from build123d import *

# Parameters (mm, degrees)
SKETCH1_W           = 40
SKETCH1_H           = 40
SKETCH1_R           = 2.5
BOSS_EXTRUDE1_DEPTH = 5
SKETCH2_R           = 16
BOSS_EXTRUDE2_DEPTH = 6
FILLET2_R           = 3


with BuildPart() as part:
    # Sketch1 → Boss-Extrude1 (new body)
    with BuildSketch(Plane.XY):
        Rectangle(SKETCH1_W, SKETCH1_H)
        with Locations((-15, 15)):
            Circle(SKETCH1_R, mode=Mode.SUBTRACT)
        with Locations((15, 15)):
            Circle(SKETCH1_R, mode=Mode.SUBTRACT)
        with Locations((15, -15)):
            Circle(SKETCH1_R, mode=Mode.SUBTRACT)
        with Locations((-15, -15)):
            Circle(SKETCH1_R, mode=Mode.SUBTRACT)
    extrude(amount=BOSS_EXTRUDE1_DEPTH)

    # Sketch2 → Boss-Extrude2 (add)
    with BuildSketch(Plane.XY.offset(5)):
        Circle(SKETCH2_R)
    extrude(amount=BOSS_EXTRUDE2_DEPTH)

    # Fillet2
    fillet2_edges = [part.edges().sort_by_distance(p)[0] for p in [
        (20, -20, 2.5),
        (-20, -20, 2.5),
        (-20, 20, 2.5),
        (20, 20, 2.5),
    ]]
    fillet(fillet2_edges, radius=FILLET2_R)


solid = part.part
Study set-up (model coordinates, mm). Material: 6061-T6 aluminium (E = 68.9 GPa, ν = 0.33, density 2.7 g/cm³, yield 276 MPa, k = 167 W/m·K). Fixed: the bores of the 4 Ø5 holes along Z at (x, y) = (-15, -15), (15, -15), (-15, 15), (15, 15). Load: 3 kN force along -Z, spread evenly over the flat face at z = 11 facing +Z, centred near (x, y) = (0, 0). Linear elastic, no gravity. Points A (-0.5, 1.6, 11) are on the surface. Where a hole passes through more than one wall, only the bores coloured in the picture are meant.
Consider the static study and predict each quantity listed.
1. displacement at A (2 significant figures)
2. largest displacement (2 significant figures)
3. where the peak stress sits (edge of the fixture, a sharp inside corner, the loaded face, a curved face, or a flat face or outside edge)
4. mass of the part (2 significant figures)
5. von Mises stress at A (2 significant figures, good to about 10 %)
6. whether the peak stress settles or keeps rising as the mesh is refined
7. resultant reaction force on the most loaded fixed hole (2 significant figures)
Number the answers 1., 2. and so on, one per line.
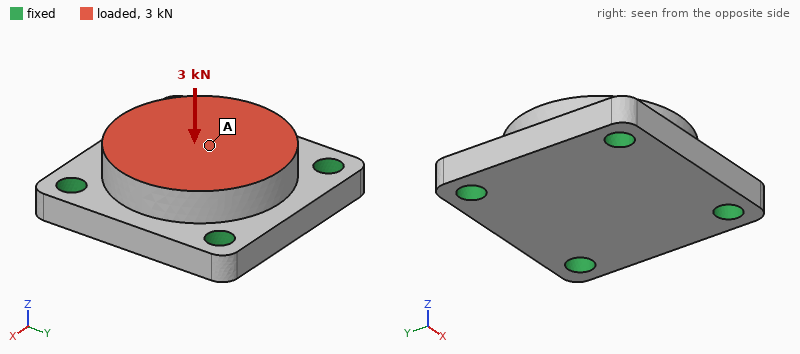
1. 6.9 µm
2. 7.0 µm
3. edge of the fixture
4. 33 g
5. 7.2 MPa
6. keeps rising
7. 820 N
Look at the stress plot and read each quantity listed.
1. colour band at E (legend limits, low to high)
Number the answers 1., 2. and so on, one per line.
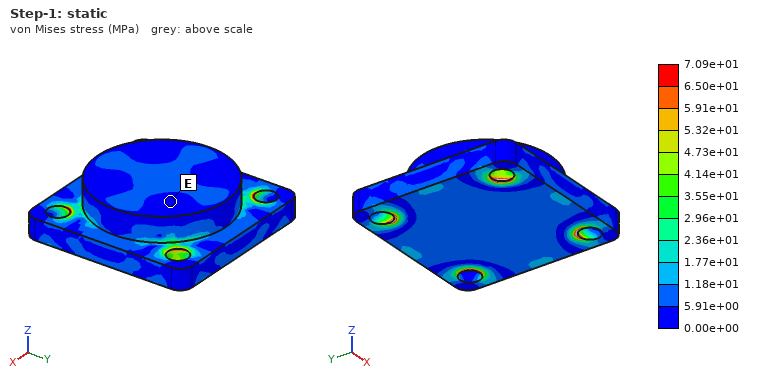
1. 0.00e+00 to 5.91e+00 MPa
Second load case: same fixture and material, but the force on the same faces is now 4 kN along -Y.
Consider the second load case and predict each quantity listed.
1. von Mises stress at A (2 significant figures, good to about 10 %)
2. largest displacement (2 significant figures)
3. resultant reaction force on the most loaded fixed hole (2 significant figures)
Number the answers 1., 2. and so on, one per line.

1. 8.6 MPa
2. 9.3 µm
3. 1.2 kN
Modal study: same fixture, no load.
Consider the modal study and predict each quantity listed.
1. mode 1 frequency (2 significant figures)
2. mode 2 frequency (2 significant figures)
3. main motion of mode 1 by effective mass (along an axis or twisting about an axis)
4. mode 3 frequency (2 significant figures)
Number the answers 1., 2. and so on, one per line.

1. 22 kHz
2. 30 kHz
3. along Z
4. 30 kHz
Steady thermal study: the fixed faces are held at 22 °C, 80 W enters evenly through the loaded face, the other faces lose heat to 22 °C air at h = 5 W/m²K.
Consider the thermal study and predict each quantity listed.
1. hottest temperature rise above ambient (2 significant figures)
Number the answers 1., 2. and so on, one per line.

1. 16 K
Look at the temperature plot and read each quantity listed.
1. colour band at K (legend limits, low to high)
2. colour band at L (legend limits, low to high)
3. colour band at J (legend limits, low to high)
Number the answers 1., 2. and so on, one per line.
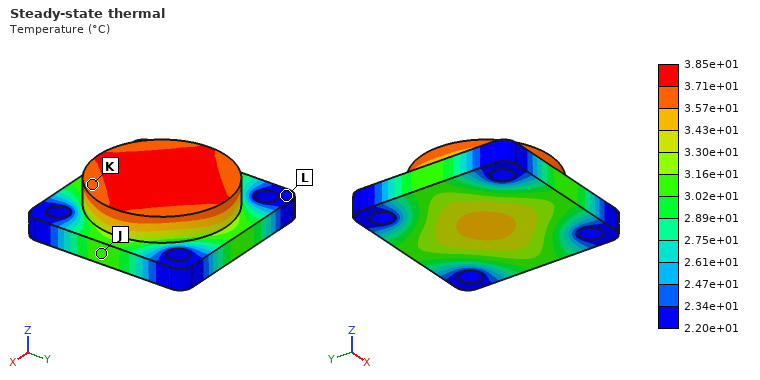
1. 3.57e+01 to 3.71e+01 °C
2. 2.20e+01 to 2.34e+01 °C
3. 3.02e+01 to 3.16e+01 °C
